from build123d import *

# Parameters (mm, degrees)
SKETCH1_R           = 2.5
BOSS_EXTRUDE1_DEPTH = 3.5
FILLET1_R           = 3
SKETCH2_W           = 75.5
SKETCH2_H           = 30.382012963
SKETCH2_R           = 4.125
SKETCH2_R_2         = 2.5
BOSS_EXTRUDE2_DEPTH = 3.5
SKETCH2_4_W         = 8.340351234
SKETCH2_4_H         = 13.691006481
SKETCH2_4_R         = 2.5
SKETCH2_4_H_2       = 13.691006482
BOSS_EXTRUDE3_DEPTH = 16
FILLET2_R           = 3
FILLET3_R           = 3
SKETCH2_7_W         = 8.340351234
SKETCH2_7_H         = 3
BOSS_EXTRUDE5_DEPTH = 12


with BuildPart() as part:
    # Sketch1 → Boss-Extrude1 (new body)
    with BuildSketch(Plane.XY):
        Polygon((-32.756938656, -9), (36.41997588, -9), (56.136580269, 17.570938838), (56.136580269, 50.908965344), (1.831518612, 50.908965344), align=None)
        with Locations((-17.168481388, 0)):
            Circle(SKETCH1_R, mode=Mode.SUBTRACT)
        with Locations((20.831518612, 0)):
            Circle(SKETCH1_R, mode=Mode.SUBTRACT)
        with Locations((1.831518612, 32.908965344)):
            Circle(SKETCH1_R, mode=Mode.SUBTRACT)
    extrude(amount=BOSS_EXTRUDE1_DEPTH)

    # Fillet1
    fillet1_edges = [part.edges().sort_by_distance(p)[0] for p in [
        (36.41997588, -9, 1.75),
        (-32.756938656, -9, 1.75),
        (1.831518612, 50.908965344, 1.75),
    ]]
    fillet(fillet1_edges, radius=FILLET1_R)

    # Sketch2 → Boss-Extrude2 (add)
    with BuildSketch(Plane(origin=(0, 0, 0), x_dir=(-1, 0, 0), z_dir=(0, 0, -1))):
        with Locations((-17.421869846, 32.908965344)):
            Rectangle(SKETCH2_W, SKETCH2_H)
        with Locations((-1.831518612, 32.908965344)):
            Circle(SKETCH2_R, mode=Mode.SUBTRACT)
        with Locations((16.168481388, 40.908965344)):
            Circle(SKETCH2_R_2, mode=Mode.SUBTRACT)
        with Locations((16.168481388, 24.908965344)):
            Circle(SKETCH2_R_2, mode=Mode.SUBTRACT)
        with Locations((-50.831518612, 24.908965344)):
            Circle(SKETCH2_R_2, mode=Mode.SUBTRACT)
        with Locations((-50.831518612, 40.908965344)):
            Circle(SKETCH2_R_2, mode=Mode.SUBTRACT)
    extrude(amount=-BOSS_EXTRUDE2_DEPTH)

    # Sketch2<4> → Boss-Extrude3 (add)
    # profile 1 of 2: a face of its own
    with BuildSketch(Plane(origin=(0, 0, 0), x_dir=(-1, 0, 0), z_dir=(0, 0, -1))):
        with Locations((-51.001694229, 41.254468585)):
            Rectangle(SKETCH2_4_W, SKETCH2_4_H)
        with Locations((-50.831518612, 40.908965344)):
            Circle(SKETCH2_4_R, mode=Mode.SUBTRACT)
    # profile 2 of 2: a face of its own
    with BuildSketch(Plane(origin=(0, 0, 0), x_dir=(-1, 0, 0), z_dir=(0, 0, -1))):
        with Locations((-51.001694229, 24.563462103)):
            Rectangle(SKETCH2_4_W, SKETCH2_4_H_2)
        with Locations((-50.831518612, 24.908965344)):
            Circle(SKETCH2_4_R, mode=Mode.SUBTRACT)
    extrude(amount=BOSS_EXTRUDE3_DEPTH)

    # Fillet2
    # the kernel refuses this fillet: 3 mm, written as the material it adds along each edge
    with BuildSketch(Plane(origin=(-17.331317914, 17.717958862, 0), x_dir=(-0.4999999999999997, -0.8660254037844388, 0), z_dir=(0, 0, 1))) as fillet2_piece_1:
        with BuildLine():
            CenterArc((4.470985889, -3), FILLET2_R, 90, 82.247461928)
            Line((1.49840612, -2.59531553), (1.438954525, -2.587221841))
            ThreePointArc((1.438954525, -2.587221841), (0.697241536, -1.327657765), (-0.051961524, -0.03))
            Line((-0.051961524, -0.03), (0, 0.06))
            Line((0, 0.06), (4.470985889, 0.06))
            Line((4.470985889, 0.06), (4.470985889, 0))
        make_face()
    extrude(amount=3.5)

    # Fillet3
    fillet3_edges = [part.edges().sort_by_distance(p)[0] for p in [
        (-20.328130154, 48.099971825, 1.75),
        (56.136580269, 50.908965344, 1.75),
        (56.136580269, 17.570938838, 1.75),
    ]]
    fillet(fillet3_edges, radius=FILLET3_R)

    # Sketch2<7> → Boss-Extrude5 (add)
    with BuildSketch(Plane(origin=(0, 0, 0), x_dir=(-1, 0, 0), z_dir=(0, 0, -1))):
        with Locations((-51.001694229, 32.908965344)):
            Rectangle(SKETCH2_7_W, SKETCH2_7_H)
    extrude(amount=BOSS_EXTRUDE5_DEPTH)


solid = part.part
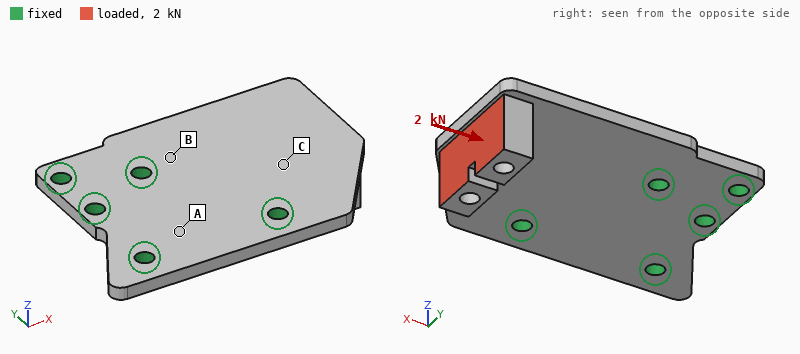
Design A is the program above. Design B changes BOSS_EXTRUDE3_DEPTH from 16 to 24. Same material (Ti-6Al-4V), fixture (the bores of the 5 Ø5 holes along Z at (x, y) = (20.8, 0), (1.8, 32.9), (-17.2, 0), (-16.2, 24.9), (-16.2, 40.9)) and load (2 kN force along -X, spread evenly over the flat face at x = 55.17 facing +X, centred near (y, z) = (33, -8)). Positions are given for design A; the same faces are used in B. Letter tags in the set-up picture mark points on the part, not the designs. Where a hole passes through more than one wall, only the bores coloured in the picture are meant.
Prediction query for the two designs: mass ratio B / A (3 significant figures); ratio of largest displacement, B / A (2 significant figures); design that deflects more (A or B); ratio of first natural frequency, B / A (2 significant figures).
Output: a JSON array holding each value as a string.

["1.08", "1.6", "B", "0.85"]
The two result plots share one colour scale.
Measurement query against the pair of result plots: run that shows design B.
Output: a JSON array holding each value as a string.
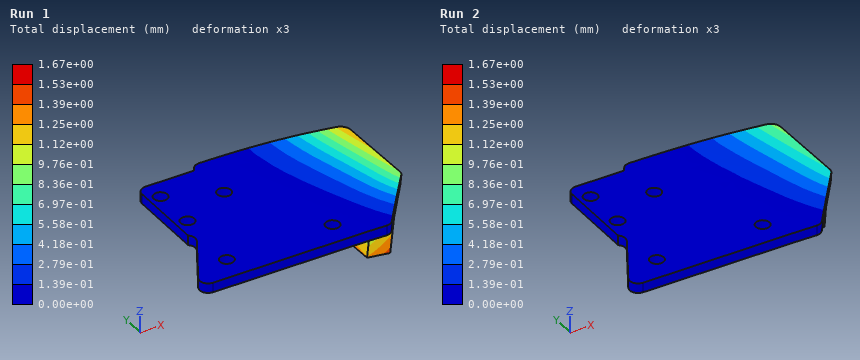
["Run 1"]
